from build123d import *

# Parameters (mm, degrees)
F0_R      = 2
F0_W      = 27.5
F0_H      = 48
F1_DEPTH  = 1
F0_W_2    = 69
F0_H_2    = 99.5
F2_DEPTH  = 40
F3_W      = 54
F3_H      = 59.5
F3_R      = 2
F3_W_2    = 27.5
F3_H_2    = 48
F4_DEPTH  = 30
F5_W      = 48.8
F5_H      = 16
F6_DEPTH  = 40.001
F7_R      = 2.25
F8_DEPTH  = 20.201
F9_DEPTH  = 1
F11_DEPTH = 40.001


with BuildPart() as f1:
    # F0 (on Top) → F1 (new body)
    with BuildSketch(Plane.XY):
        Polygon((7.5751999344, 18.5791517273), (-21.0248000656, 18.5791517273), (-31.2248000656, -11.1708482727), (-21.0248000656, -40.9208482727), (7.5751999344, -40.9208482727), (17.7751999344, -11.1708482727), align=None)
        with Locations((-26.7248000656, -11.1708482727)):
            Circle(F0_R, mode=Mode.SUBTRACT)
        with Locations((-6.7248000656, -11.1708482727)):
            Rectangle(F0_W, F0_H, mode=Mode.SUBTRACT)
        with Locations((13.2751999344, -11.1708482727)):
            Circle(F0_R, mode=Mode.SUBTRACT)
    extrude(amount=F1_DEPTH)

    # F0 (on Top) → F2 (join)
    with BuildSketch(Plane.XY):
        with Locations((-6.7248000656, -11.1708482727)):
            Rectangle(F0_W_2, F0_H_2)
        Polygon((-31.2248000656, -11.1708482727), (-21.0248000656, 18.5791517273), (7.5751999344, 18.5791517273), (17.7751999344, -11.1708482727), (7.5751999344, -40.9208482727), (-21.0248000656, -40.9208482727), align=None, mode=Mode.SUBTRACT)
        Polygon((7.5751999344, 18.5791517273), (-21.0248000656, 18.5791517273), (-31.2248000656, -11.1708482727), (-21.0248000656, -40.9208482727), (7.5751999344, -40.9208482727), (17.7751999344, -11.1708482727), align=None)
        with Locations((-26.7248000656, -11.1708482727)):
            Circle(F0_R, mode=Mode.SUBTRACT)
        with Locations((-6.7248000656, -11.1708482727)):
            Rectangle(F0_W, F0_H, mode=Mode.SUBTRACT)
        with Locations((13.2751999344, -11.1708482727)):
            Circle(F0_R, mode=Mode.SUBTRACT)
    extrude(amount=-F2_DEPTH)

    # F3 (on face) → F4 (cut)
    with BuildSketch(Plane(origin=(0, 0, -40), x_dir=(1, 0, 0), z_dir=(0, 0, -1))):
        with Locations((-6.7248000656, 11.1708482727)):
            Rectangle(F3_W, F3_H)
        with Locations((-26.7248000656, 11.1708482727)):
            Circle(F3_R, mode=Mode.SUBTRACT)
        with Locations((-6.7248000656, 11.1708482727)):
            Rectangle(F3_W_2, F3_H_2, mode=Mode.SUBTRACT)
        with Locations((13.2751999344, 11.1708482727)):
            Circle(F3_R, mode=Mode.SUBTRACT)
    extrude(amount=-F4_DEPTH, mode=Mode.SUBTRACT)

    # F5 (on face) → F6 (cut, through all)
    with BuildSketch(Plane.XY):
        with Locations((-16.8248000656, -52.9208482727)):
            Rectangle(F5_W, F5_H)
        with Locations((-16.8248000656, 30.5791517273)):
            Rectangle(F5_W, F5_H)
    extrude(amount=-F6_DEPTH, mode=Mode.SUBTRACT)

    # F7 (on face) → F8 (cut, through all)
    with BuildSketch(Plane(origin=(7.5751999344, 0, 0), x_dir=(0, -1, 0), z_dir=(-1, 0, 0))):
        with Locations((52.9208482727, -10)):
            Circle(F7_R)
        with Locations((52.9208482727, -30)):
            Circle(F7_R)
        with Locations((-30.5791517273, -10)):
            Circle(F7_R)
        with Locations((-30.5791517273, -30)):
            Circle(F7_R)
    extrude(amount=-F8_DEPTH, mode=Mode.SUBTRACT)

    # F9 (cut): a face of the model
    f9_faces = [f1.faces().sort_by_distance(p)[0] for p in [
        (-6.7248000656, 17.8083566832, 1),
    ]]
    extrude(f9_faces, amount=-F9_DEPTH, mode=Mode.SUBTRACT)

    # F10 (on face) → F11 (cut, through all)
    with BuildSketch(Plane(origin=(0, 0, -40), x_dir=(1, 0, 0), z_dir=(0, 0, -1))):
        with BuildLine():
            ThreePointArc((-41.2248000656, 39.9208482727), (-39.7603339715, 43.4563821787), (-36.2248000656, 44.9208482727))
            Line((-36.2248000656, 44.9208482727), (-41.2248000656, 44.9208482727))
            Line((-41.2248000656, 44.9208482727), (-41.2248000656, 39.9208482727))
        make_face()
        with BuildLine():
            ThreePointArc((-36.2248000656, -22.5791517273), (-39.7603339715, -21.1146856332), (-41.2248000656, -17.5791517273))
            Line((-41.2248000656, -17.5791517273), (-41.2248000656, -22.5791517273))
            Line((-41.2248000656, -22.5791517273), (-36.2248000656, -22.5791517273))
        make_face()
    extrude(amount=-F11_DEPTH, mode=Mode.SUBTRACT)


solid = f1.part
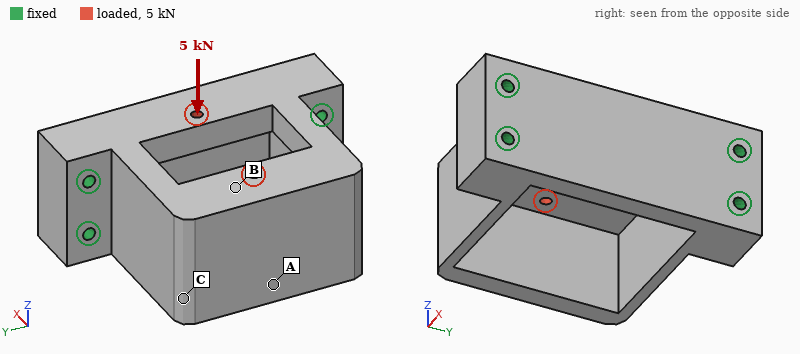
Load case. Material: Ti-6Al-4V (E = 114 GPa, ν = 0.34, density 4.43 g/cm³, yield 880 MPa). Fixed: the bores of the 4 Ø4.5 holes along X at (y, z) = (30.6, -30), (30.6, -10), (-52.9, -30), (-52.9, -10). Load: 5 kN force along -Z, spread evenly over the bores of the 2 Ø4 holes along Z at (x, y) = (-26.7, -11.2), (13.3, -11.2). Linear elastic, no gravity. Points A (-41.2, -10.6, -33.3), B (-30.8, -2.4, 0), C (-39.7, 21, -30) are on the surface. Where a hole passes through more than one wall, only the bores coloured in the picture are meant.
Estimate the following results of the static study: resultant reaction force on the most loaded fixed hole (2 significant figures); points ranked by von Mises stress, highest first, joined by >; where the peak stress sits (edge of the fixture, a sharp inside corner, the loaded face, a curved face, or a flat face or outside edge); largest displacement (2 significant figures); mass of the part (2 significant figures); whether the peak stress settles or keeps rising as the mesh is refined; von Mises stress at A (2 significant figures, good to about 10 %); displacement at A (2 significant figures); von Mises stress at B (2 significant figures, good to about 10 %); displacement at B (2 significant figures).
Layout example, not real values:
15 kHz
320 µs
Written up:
2.7 kN
B > A > C
a sharp inside corner
40 µm
450 g
keeps rising
13 MPa
34 µm
28 MPa
34 µm
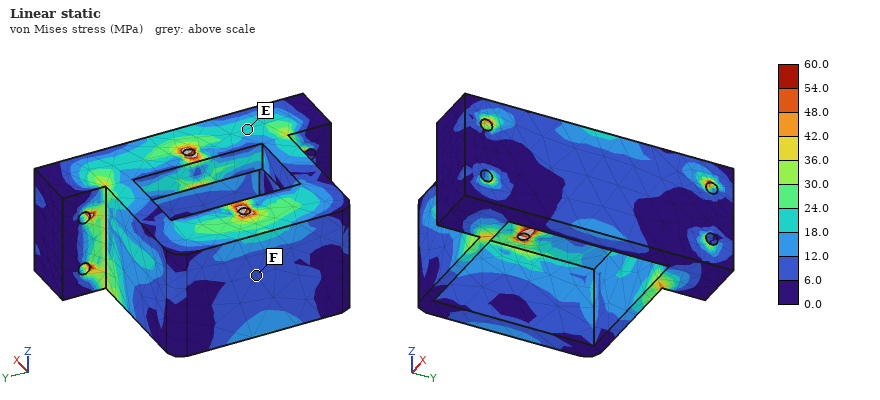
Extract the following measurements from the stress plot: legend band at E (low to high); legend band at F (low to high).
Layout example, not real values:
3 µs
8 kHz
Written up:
18.0 to 24.0 MPa
6.0 to 12.0 MPa
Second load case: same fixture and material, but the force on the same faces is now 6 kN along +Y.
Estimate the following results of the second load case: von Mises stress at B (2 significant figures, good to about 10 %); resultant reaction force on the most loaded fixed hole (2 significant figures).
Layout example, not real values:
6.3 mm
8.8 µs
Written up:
13 MPa
2.9 kN
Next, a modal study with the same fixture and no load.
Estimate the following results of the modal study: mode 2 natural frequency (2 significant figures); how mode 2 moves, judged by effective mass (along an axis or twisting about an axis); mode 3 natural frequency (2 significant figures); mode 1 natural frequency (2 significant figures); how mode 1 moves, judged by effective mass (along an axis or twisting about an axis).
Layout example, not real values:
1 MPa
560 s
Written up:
3600 Hz
along Z
5700 Hz
2500 Hz
along Y
